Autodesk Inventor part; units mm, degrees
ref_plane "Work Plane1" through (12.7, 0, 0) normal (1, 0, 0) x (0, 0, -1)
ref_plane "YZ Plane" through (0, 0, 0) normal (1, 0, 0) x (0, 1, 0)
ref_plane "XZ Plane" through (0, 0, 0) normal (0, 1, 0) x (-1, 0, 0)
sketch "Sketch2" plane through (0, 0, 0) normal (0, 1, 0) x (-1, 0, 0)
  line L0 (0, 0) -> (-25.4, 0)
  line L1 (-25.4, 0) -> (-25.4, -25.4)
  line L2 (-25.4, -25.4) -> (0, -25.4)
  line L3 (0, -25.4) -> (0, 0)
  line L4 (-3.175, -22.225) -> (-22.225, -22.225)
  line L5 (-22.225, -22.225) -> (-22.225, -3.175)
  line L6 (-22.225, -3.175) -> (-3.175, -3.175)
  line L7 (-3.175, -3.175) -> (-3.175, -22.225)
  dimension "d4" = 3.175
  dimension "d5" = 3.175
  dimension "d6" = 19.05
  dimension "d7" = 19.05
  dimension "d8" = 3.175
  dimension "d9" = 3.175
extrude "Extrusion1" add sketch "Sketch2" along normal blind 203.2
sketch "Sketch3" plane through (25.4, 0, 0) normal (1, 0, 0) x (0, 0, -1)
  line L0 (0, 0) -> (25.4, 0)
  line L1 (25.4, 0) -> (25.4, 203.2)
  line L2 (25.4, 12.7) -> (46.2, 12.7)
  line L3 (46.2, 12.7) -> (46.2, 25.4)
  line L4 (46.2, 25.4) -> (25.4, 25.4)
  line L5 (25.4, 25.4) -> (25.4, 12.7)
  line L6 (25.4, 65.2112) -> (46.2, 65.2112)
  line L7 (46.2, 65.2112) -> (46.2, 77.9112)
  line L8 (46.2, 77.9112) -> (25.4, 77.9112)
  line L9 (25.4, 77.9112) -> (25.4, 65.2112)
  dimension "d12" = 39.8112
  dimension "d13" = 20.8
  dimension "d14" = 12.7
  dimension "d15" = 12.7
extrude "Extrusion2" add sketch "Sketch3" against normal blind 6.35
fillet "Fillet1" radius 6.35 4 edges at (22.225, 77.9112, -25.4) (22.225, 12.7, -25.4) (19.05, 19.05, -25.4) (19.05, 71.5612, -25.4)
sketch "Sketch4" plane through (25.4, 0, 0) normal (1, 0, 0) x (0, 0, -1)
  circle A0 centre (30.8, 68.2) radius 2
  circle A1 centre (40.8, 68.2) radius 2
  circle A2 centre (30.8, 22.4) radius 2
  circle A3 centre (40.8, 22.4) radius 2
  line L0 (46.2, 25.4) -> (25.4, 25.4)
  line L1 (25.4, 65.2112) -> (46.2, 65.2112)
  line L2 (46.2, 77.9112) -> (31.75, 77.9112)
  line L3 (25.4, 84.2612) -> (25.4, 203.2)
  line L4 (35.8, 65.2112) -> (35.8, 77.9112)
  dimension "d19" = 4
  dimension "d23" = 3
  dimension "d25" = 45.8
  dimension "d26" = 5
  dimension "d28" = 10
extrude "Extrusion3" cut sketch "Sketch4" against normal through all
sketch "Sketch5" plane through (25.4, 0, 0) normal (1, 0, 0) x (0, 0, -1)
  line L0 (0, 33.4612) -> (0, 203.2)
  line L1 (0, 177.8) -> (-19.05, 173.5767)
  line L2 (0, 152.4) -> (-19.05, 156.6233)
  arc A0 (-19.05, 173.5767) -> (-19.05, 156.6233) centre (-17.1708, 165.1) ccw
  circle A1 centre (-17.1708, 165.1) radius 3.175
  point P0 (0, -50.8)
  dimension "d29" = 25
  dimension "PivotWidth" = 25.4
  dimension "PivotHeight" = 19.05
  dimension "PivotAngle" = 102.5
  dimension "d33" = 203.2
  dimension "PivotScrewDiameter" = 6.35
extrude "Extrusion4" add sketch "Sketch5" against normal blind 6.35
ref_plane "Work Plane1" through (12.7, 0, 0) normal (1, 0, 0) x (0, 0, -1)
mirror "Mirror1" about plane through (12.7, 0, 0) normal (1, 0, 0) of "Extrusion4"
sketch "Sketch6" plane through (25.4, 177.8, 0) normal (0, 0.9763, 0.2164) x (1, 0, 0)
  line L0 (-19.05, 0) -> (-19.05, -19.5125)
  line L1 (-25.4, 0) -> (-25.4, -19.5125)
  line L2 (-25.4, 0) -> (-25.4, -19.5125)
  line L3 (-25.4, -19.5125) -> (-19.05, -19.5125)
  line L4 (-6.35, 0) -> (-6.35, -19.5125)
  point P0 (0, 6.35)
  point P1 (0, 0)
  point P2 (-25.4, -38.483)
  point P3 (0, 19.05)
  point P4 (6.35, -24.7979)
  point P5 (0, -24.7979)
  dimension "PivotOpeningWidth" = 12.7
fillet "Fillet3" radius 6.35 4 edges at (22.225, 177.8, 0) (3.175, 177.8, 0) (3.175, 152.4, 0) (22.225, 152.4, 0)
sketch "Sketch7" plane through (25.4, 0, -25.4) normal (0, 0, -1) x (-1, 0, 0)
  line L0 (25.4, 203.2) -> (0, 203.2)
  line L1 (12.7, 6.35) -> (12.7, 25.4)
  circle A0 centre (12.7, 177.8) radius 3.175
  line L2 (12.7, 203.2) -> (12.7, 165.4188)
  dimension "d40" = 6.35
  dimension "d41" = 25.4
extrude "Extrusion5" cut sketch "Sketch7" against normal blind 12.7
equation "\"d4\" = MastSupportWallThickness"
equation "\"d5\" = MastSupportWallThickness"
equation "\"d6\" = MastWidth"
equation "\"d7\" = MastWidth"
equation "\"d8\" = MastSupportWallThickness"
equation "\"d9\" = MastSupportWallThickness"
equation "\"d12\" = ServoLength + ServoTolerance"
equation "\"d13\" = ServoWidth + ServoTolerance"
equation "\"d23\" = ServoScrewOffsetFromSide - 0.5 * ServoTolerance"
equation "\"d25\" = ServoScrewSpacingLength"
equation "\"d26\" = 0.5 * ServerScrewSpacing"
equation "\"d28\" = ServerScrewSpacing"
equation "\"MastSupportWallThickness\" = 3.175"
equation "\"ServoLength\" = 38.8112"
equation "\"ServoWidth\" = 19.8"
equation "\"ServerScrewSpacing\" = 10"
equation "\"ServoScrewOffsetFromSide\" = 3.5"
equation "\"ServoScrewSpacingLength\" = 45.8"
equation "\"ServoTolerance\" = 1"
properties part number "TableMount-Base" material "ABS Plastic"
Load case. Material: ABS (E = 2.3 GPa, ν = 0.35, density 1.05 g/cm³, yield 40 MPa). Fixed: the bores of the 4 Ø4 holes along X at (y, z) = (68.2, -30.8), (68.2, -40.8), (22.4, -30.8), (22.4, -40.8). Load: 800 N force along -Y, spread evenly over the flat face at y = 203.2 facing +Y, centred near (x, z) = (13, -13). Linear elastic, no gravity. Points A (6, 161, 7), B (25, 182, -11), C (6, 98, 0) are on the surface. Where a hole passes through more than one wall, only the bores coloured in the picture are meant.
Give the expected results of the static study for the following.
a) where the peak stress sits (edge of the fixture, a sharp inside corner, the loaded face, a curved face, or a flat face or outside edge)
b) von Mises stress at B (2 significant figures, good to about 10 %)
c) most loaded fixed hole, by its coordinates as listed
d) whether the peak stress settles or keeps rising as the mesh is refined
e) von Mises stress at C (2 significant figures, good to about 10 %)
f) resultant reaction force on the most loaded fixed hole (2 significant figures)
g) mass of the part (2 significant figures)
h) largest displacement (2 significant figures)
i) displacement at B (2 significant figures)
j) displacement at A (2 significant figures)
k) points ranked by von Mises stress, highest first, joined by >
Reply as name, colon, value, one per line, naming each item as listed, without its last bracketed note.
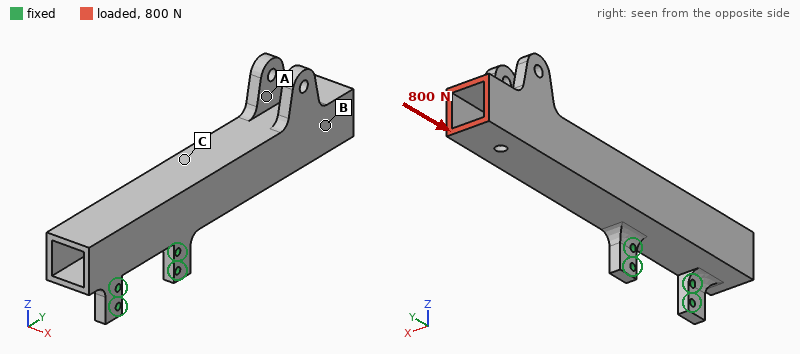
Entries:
where the peak stress sits: edge of the fixture
von Mises stress at B: 2.6 MPa
most loaded fixed hole, by its coordinates as listed: (68.2, -30.8)
whether the peak stress settles or keeps rising as the mesh is refined: keeps rising
von Mises stress at C: 3.3 MPa
resultant reaction force on the most loaded fixed hole: 590 N
mass of the part: 70 g
largest displacement: 0.90 mm
displacement at B: 0.73 mm
displacement at A: 0.69 mm
points ranked by von Mises stress, highest first, joined by >: C > B > A
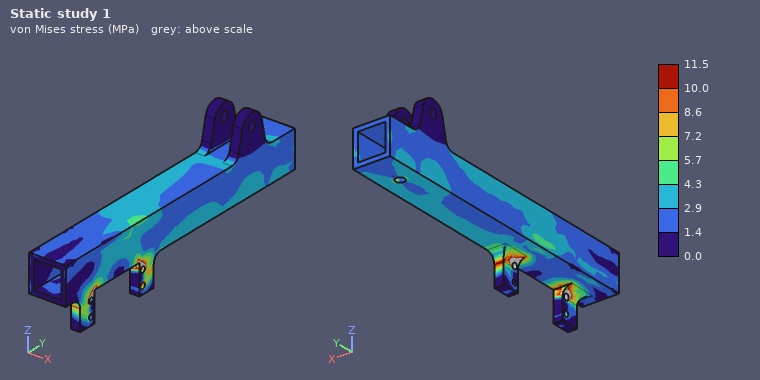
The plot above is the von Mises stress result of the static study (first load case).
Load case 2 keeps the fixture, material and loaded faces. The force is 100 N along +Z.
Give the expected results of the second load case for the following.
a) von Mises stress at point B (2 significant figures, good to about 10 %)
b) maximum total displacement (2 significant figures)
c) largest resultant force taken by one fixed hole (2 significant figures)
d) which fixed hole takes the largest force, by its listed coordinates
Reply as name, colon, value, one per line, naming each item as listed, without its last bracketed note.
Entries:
von Mises stress at point B: 1.3 MPa
maximum total displacement: 2.6 mm
largest resultant force taken by one fixed hole: 270 N
which fixed hole takes the largest force, by its listed coordinates: (22.4, -30.8)
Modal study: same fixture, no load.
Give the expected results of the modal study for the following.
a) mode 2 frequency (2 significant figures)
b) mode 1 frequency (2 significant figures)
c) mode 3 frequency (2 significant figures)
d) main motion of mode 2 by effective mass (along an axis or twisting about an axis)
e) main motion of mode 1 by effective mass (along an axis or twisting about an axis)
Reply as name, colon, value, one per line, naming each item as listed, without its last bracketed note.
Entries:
mode 2 frequency: 270 Hz
mode 1 frequency: 210 Hz
mode 3 frequency: 450 Hz
main motion of mode 2 by effective mass: along Z
main motion of mode 1 by effective mass: along X
